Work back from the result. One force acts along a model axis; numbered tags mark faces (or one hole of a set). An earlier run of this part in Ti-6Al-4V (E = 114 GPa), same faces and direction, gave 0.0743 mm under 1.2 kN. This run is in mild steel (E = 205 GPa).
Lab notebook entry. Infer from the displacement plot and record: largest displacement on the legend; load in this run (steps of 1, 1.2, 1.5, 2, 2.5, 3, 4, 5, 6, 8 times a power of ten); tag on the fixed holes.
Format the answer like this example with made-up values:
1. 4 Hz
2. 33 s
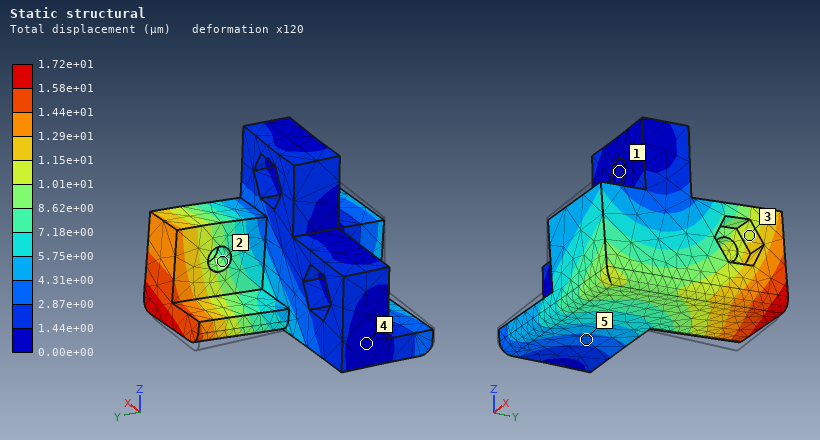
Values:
1. 1.72e+01 µm
2. 500 N
3. 1
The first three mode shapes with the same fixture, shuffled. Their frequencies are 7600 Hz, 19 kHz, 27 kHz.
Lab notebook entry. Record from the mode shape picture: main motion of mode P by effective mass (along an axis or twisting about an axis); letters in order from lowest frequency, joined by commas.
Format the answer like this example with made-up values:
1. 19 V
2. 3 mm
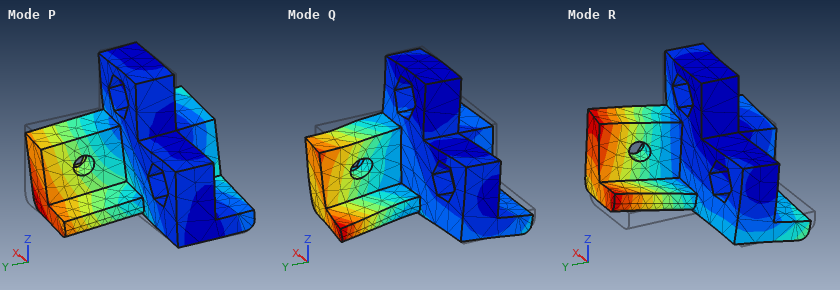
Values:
1. along Y
2. P, R, Q
